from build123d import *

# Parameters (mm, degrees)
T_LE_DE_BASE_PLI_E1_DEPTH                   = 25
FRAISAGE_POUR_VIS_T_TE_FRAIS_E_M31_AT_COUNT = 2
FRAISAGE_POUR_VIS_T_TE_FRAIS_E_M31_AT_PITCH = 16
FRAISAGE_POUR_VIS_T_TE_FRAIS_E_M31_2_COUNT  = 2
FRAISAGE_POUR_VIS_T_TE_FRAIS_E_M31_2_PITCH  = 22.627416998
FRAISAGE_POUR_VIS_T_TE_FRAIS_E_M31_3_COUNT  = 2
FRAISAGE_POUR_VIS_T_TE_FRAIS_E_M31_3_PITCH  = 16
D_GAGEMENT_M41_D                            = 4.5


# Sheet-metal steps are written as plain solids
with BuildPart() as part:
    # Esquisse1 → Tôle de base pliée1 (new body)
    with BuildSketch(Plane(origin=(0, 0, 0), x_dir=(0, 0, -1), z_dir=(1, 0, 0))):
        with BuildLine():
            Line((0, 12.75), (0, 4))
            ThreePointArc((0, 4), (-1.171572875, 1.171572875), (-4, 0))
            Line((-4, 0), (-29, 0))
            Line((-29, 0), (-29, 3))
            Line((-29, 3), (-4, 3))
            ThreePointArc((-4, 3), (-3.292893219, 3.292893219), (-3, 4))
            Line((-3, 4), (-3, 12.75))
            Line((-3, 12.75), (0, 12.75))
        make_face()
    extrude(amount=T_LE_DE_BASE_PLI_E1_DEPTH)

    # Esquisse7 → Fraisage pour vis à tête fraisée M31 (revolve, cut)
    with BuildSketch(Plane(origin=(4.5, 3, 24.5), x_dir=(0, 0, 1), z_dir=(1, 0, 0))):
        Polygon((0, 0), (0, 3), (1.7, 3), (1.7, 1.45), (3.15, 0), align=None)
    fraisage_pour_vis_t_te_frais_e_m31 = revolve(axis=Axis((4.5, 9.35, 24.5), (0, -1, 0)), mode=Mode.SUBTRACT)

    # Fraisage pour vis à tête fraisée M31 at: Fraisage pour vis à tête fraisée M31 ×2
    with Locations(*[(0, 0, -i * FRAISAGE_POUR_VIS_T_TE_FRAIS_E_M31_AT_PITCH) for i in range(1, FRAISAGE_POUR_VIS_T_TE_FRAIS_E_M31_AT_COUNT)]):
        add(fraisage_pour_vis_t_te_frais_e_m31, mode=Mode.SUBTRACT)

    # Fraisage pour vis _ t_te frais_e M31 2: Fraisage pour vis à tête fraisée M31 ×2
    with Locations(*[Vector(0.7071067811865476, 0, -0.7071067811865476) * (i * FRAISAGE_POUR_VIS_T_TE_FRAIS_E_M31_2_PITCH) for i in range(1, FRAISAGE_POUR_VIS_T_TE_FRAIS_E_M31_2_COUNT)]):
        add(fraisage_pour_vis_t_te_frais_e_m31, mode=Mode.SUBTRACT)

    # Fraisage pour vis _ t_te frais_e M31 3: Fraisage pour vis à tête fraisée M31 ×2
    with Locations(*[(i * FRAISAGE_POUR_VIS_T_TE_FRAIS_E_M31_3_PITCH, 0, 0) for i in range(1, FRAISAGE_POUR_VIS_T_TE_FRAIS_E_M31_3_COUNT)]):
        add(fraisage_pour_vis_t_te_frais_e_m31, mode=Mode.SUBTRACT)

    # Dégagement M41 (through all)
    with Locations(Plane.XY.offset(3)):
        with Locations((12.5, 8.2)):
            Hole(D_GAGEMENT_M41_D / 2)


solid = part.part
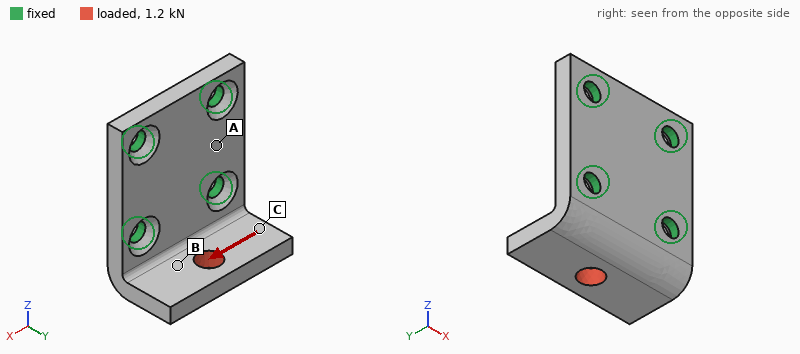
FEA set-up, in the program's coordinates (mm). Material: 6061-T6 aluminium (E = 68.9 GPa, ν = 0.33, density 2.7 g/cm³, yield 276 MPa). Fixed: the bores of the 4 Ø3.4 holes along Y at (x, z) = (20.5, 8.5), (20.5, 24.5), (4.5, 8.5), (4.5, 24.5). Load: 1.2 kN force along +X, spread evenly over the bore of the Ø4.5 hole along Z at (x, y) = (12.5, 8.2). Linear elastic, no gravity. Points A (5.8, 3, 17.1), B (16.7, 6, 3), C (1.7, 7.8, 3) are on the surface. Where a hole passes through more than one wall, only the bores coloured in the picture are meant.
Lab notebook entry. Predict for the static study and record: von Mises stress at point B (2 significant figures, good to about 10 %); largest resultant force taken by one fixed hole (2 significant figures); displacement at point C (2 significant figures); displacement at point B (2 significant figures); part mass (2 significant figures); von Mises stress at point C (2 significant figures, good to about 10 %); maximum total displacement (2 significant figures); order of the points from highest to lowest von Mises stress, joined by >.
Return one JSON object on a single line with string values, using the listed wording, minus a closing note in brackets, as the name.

{"von Mises stress at point B": "65 MPa", "largest resultant force taken by one fixed hole": "910 N", "displacement at point C": "42 µm", "displacement at point B": "23 µm", "part mass": "7.1 g", "von Mises stress at point C": "34 MPa", "maximum total displacement": "63 µm", "order of the points from highest to lowest von Mises stress, joined by >": "B > C > A"}
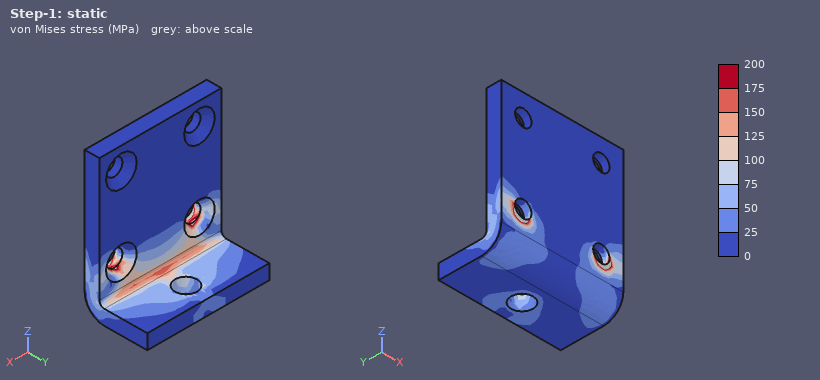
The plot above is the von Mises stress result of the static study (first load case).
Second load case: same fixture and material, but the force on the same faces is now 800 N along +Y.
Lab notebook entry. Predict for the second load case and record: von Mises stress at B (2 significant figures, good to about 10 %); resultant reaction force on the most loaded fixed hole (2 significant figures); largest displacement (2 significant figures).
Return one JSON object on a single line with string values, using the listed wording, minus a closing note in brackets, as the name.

{"von Mises stress at B": "21 MPa", "resultant reaction force on the most loaded fixed hole": "510 N", "largest displacement": "99 µm"}
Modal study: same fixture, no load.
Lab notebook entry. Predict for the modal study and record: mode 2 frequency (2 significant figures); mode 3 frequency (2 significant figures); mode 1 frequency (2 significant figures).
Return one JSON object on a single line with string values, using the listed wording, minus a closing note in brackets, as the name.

{"mode 2 frequency": "14 kHz", "mode 3 frequency": "26 kHz", "mode 1 frequency": "8800 Hz"}
